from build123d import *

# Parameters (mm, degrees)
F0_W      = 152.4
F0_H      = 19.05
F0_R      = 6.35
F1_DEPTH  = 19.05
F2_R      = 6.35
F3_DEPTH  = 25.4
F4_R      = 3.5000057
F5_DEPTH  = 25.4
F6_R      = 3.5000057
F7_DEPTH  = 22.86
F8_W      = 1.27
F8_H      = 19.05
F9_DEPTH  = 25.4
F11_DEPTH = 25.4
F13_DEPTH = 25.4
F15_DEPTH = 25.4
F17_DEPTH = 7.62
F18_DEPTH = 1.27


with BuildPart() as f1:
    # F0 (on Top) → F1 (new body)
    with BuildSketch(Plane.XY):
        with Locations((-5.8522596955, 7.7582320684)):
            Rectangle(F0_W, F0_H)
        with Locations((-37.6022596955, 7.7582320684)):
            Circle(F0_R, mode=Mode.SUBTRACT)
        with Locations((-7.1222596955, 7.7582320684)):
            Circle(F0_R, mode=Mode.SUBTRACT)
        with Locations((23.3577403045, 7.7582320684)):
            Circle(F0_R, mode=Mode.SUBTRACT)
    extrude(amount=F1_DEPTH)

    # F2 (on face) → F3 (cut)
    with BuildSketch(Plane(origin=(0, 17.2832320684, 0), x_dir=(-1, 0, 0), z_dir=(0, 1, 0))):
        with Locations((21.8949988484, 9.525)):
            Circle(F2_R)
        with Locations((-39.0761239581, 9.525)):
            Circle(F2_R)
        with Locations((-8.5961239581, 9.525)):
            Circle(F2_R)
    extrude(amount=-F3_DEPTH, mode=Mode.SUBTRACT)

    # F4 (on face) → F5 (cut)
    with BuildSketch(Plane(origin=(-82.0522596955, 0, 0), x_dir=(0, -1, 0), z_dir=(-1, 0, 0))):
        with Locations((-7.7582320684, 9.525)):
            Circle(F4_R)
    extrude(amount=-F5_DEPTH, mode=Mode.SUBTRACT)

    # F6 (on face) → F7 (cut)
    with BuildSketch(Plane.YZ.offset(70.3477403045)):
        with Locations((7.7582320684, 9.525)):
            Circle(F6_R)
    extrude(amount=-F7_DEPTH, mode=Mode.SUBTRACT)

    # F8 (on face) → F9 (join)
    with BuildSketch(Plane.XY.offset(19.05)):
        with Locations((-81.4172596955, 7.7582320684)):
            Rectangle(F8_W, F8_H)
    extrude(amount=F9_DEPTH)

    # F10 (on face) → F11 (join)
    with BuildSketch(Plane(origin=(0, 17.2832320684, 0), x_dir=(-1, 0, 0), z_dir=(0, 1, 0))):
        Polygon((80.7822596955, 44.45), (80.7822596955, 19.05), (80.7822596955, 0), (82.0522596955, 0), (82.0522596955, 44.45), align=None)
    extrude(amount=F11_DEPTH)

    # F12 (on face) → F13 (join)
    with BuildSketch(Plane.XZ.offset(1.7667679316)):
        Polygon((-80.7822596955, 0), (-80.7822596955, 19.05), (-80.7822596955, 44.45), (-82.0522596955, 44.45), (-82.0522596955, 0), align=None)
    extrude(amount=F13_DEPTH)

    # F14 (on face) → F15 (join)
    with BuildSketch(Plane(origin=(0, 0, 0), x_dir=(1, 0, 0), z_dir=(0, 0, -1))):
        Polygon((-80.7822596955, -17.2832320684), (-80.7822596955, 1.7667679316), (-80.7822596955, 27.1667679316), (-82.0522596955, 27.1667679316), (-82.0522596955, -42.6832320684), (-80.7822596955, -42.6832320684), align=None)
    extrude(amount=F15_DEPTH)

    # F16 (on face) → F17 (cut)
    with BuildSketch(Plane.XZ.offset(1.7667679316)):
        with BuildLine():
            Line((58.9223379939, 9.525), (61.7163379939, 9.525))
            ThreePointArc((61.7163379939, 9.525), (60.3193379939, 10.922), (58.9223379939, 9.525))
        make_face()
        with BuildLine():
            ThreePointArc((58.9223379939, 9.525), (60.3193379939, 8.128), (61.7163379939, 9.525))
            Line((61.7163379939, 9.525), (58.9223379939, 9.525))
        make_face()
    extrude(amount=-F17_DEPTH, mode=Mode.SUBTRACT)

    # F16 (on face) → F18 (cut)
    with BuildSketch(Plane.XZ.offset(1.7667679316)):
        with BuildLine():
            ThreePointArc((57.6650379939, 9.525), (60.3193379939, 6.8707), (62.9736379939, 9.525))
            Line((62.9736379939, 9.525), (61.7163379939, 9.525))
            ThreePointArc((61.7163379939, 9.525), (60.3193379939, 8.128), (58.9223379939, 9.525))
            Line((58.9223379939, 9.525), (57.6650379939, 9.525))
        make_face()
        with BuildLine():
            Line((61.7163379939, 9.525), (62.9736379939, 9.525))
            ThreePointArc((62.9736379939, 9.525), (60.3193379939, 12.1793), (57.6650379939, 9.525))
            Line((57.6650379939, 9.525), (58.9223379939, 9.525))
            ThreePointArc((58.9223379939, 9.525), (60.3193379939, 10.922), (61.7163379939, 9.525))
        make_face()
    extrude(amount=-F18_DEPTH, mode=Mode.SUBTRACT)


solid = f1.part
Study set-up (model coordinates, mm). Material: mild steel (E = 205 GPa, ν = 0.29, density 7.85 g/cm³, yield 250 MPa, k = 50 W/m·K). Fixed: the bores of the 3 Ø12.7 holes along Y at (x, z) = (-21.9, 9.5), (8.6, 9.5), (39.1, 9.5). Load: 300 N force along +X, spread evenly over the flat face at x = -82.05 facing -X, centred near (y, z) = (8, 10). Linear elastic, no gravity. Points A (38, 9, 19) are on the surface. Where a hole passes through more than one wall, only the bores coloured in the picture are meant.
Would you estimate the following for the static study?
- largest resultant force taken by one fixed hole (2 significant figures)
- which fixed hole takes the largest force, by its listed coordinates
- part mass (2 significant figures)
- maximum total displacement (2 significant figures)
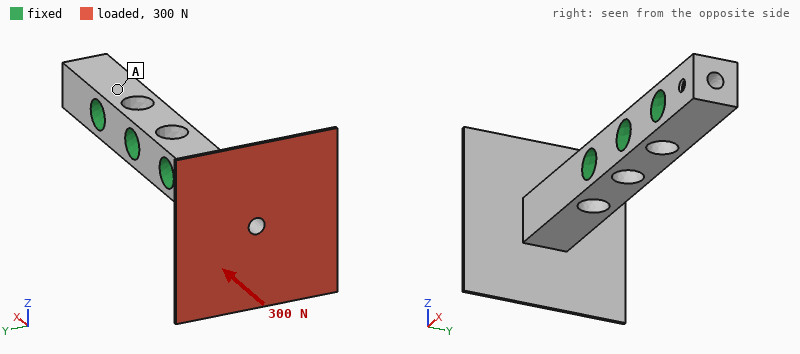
300 N
(-21.9, 9.5)
350 g
0.23 mm
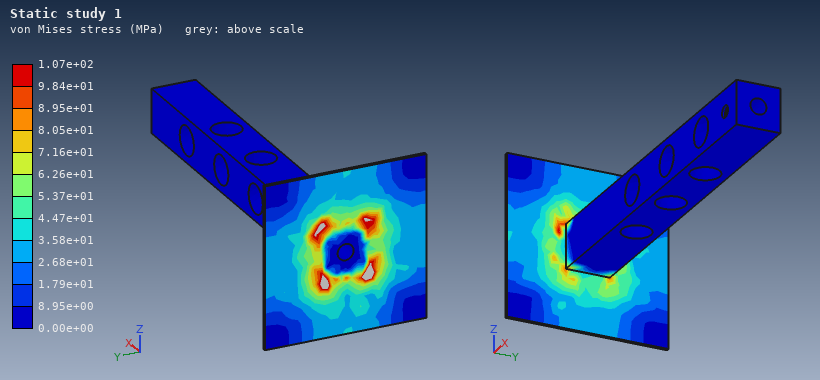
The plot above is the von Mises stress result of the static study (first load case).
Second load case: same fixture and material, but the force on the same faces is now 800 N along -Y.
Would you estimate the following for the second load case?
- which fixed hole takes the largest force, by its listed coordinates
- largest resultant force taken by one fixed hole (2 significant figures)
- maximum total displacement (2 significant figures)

(-21.9, 9.5)
800 N
62 µm
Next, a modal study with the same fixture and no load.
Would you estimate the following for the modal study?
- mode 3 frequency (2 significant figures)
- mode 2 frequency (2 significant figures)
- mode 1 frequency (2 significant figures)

1200 Hz
1100 Hz
1100 Hz
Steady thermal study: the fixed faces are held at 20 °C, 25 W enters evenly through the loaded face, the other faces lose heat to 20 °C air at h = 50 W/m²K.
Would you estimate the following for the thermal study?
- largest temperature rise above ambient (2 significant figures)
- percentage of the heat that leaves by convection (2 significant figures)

60 K
73 %
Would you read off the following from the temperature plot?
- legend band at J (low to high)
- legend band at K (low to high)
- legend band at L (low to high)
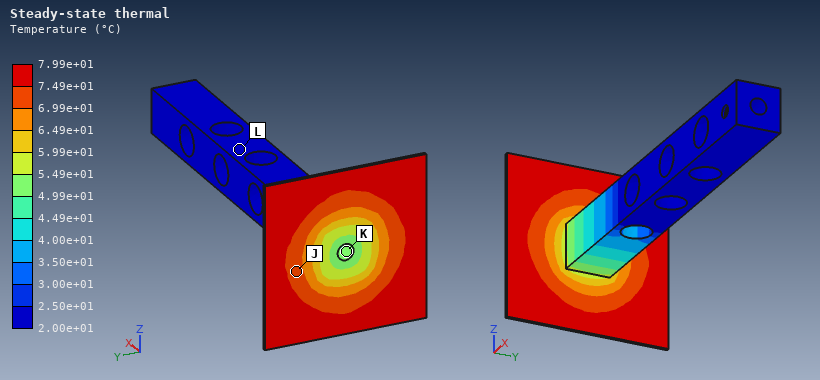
6.99e+01 to 7.49e+01 °C
4.99e+01 to 5.49e+01 °C
2.00e+01 to 2.50e+01 °C
